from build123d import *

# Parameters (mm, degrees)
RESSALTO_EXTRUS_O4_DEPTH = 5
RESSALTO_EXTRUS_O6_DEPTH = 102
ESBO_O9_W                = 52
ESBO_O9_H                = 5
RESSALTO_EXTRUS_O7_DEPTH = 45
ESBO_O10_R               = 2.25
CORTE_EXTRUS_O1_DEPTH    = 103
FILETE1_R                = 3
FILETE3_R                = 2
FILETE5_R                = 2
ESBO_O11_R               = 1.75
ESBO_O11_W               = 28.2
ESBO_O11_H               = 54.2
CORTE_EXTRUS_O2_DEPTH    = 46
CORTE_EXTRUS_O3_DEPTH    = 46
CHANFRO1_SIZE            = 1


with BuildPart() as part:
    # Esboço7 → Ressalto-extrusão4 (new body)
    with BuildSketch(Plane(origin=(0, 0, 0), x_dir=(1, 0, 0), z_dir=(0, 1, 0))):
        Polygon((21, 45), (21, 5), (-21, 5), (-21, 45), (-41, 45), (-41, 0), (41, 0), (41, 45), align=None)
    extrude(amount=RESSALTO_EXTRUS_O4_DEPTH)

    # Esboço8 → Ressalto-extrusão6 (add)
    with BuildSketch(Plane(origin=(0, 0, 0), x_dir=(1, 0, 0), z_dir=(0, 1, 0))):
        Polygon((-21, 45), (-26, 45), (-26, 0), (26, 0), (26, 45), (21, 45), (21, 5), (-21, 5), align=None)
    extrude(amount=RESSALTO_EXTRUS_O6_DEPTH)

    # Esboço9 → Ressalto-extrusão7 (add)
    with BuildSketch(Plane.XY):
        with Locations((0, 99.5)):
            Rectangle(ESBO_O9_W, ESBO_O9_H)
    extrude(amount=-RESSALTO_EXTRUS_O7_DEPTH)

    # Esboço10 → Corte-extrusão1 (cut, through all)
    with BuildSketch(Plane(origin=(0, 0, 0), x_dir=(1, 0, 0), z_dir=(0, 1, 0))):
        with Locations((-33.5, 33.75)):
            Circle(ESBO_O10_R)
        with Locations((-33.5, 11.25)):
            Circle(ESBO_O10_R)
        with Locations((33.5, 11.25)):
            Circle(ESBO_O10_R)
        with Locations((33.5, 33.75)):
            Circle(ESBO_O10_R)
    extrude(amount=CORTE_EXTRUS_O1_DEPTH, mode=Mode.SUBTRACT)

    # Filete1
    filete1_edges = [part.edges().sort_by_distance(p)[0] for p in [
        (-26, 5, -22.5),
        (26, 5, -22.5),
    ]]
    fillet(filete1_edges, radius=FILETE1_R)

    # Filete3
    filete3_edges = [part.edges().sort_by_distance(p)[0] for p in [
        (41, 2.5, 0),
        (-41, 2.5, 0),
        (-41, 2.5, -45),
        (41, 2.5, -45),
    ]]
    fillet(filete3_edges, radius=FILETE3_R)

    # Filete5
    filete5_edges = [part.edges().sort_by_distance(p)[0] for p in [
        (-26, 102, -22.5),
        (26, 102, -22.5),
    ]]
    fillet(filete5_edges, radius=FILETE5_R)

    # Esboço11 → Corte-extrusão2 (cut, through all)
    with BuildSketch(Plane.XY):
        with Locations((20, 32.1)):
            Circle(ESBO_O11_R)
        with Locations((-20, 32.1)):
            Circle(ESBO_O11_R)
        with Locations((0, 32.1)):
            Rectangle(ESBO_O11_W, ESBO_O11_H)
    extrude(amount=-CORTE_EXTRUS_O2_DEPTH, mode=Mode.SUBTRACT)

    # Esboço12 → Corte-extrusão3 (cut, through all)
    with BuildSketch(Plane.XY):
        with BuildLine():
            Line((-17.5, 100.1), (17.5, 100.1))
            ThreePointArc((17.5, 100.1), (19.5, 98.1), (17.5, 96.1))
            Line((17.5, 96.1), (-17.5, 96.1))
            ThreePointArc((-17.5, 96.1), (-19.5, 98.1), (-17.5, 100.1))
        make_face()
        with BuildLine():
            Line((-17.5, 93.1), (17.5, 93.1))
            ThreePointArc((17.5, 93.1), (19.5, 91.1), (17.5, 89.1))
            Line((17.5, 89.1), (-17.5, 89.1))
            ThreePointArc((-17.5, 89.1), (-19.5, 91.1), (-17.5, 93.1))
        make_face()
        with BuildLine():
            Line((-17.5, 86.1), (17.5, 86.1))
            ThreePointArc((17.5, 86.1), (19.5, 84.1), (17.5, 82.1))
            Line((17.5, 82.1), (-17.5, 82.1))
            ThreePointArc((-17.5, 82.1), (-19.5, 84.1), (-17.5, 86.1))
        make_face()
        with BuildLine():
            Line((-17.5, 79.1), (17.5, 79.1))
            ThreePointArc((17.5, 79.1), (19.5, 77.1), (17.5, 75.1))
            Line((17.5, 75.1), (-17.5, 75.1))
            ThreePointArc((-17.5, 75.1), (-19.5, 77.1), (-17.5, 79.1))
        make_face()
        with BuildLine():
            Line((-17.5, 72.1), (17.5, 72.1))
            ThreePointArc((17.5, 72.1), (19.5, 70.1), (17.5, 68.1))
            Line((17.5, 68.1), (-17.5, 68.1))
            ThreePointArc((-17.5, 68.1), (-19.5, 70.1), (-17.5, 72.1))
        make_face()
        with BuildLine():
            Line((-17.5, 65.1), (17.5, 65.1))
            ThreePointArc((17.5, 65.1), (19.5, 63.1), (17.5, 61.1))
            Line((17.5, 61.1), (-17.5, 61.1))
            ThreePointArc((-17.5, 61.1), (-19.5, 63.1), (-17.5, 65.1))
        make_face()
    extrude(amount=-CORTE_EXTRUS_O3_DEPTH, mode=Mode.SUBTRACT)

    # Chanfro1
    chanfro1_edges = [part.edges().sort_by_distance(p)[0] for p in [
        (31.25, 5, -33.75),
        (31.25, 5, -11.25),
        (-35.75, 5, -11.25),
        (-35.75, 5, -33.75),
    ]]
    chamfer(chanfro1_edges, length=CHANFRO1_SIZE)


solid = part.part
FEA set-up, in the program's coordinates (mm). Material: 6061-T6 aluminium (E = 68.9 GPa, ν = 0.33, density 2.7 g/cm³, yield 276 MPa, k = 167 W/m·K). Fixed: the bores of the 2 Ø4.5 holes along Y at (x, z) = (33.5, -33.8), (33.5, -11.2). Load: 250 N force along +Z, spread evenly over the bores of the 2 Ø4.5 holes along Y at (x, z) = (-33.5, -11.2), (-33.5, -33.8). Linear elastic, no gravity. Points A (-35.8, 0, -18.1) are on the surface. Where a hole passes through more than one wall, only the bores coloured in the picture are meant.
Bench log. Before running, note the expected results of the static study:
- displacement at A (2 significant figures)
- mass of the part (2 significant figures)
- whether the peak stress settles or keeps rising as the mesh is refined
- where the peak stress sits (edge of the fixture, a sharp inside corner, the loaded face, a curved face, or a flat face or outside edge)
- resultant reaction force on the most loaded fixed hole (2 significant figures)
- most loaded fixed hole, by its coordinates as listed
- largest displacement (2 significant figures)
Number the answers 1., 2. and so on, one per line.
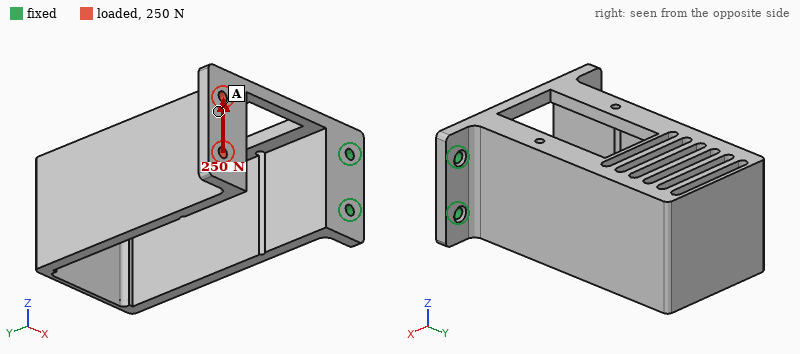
1. 1.2 mm
2. 180 g
3. keeps rising
4. a sharp inside corner
5. 680 N
6. (33.5, -33.8)
7. 1.5 mm
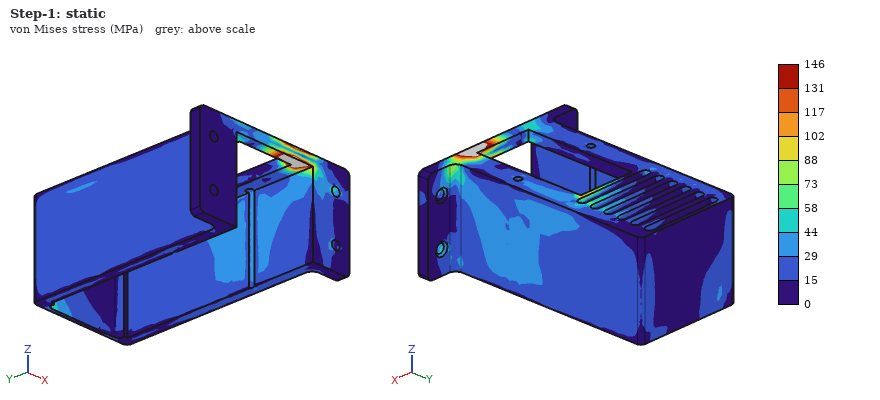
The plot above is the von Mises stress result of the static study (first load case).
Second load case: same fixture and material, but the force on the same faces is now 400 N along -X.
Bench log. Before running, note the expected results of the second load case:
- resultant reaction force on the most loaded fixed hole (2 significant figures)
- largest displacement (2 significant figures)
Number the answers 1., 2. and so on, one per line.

1. 210 N
2. 1.2 mm
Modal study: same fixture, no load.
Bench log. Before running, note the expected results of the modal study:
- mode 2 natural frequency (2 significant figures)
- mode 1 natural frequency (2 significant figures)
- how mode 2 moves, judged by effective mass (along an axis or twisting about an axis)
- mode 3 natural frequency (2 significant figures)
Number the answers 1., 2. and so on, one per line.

1. 320 Hz
2. 230 Hz
3. along Z
4. 690 Hz
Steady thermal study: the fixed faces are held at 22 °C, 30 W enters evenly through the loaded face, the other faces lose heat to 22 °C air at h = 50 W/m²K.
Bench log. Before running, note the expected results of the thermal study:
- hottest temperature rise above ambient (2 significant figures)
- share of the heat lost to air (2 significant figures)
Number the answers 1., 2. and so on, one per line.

1. 53 K
2. 82 %
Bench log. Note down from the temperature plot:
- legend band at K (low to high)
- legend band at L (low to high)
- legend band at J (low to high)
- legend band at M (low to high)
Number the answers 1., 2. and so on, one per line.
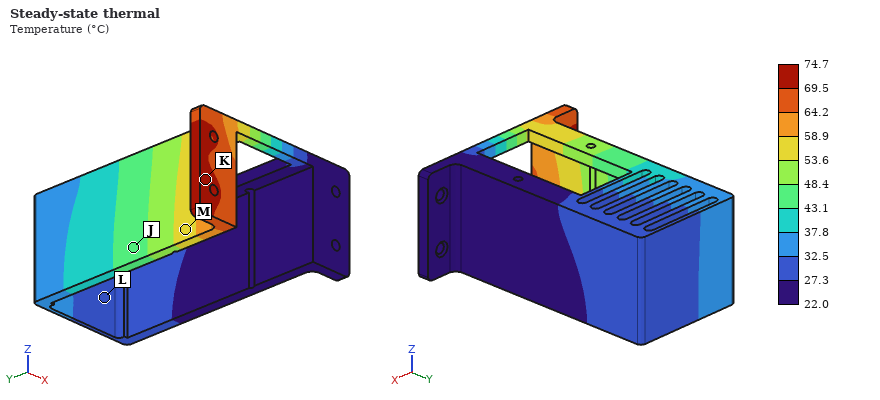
1. 69.5 to 74.7 °C
2. 27.3 to 32.5 °C
3. 43.1 to 48.4 °C
4. 53.6 to 58.9 °C
